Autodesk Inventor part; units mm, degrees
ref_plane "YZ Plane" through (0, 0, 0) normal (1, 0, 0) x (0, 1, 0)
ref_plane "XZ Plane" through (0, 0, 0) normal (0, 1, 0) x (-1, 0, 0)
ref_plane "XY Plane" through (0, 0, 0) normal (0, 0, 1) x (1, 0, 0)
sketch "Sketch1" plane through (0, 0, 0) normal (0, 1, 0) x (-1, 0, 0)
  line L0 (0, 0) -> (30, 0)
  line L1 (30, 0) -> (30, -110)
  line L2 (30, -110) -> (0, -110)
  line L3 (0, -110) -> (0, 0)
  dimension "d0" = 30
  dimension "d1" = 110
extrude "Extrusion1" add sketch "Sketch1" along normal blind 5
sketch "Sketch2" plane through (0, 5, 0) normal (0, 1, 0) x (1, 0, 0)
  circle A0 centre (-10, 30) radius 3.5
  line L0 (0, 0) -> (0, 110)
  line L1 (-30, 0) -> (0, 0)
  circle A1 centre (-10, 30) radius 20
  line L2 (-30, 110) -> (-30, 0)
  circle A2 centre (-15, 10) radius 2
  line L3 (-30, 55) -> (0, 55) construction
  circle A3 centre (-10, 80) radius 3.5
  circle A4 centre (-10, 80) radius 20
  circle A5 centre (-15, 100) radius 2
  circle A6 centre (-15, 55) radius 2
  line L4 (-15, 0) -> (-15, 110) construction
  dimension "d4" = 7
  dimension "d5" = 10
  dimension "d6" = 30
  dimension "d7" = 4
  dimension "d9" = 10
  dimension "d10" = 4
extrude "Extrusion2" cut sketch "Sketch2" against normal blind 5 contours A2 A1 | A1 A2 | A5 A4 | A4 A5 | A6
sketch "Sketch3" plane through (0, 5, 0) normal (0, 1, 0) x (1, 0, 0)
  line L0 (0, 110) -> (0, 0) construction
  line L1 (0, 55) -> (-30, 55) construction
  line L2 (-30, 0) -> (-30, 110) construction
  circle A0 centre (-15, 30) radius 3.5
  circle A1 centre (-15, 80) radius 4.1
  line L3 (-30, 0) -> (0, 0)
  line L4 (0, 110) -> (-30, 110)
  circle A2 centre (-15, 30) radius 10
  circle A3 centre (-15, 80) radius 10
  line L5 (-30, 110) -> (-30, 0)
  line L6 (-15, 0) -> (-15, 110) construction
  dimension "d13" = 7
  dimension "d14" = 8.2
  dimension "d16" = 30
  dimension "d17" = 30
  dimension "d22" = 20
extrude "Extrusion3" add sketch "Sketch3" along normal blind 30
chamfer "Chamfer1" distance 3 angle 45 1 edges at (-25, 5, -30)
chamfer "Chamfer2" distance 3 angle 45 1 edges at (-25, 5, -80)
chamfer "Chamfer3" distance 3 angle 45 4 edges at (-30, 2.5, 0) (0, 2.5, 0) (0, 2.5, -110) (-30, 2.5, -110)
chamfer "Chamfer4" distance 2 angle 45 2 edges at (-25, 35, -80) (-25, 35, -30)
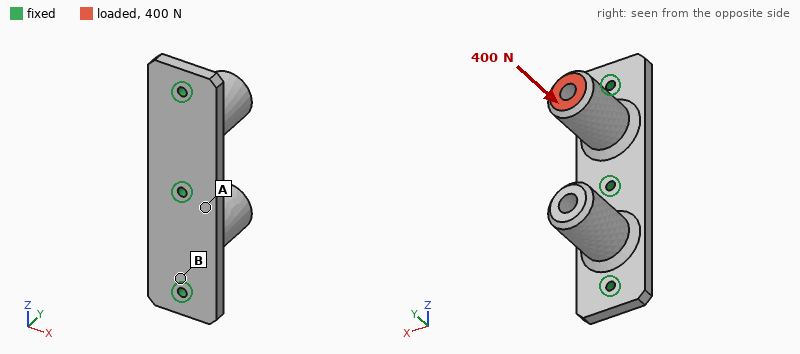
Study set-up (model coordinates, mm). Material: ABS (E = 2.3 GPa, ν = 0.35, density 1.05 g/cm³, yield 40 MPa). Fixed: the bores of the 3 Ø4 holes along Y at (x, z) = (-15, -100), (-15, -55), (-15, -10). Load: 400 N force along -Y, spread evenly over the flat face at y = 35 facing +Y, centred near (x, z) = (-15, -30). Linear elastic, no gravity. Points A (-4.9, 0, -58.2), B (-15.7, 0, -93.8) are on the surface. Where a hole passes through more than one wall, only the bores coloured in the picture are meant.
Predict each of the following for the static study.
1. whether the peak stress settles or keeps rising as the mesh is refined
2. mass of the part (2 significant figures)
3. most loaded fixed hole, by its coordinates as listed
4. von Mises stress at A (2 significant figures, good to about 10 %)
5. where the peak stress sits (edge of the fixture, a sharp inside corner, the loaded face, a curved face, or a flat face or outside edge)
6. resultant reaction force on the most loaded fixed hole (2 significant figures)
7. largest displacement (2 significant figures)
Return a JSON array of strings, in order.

["keeps rising", "34 g", "(-15, -10)", "3.2 MPa", "edge of the fixture", "240 N", "0.18 mm"]
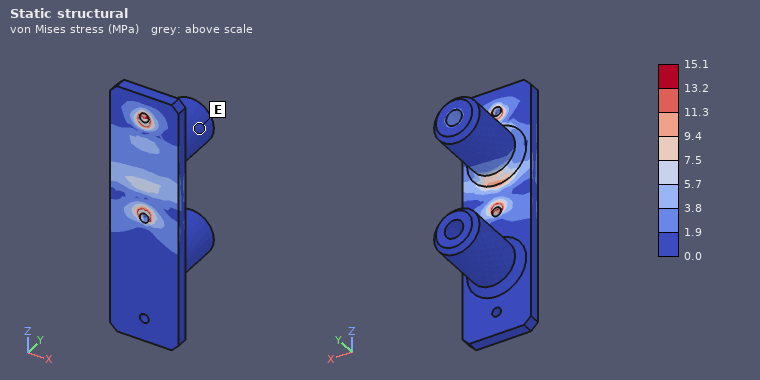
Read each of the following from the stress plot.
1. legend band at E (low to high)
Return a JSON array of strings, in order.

["0.0 to 1.9 MPa"]
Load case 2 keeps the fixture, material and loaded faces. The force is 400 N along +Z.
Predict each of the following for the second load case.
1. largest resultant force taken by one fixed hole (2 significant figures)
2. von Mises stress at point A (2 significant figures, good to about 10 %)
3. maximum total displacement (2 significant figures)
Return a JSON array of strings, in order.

["420 N", "5.0 MPa", "0.74 mm"]
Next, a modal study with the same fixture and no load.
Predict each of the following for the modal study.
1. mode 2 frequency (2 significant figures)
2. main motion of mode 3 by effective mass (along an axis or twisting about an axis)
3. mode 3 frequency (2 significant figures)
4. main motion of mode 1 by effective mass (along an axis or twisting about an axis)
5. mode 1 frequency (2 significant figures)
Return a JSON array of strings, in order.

["1000 Hz", "along Z", "2000 Hz", "along X", "950 Hz"]
